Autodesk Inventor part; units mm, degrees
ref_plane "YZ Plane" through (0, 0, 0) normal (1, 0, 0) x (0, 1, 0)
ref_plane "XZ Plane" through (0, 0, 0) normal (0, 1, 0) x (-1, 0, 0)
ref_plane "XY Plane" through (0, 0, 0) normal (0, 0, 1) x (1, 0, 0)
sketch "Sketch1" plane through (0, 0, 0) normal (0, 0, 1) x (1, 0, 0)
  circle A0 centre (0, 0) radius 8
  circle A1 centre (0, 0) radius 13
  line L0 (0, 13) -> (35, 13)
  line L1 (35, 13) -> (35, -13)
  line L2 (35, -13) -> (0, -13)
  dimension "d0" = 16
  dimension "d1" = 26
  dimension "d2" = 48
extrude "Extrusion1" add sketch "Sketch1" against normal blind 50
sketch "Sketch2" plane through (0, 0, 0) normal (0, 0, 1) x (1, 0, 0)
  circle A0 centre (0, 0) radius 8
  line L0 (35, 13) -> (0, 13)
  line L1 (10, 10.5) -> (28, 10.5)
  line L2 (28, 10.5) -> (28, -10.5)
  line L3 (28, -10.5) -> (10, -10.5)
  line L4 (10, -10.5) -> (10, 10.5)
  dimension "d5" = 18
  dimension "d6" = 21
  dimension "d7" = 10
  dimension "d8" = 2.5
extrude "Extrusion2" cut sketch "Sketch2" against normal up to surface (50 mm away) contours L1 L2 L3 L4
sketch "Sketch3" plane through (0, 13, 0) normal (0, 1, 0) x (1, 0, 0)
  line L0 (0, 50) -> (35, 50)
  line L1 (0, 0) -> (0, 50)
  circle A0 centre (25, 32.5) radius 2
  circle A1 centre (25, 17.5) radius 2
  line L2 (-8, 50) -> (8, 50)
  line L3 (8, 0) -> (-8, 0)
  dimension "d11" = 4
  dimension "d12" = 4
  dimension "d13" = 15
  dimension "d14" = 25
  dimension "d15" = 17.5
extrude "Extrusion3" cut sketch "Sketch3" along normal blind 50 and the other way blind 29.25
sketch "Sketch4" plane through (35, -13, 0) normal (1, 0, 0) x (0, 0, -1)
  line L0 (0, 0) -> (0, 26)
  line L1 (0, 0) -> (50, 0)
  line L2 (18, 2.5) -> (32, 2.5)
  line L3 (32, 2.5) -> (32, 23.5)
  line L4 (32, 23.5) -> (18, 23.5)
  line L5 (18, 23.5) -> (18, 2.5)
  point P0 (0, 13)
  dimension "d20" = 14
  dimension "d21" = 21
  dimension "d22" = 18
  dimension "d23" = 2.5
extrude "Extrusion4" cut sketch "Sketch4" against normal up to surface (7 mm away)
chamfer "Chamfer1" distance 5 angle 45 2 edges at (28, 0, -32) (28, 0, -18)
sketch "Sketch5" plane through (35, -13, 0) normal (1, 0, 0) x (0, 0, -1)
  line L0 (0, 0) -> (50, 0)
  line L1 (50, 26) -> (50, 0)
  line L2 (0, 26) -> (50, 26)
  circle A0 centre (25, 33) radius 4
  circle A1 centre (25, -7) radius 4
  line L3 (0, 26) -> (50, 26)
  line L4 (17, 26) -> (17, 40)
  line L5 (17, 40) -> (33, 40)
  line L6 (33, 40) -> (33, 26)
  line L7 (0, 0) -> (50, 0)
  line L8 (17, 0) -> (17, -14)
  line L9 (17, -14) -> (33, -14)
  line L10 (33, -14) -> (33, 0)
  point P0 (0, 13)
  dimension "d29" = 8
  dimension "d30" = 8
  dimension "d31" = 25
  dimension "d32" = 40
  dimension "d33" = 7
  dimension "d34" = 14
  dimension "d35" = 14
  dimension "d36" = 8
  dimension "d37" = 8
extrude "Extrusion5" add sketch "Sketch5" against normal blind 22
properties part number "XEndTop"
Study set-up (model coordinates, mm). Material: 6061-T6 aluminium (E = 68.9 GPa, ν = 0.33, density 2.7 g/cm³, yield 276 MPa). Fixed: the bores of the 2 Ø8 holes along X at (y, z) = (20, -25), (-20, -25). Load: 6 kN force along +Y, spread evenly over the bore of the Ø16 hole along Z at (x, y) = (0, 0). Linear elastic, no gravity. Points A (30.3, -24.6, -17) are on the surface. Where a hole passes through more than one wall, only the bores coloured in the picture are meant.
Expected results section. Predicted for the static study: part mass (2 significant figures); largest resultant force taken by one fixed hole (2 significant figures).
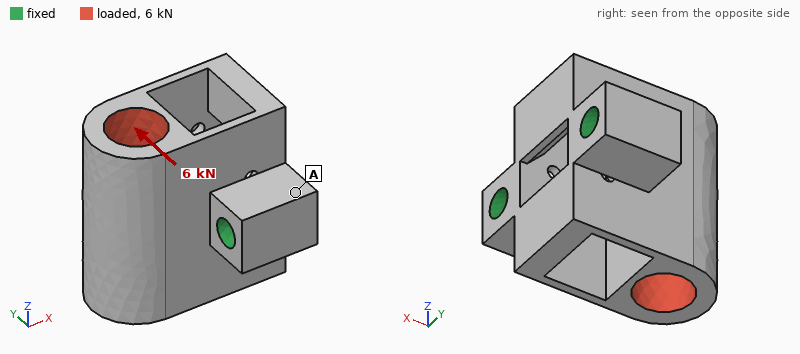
94 g
4.2 kN
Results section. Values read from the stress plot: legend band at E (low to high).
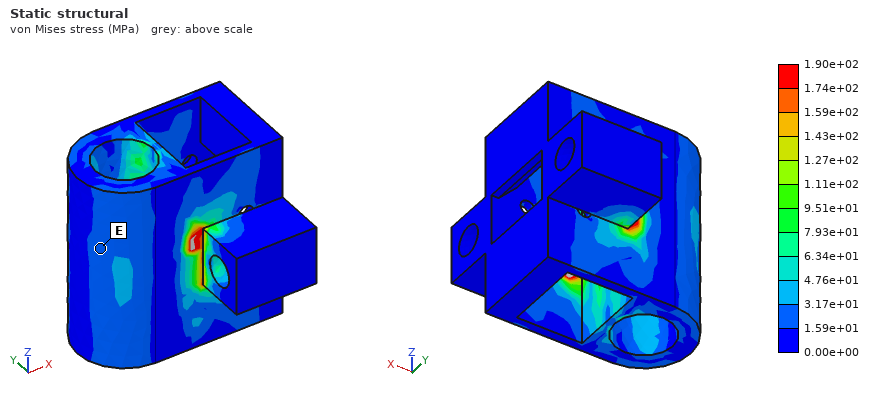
1.59e+01 to 3.17e+01 MPa
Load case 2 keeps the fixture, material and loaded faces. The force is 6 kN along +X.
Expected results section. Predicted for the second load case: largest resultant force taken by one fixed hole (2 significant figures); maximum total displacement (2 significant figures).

3.1 kN
16 µm
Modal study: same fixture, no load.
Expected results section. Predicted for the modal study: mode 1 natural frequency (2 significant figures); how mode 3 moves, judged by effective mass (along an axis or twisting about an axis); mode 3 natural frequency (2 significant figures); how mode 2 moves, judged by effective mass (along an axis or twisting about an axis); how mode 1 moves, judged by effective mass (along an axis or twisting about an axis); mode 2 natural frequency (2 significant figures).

6400 Hz
twisting about X
9400 Hz
along Y
along Z
7300 Hz
